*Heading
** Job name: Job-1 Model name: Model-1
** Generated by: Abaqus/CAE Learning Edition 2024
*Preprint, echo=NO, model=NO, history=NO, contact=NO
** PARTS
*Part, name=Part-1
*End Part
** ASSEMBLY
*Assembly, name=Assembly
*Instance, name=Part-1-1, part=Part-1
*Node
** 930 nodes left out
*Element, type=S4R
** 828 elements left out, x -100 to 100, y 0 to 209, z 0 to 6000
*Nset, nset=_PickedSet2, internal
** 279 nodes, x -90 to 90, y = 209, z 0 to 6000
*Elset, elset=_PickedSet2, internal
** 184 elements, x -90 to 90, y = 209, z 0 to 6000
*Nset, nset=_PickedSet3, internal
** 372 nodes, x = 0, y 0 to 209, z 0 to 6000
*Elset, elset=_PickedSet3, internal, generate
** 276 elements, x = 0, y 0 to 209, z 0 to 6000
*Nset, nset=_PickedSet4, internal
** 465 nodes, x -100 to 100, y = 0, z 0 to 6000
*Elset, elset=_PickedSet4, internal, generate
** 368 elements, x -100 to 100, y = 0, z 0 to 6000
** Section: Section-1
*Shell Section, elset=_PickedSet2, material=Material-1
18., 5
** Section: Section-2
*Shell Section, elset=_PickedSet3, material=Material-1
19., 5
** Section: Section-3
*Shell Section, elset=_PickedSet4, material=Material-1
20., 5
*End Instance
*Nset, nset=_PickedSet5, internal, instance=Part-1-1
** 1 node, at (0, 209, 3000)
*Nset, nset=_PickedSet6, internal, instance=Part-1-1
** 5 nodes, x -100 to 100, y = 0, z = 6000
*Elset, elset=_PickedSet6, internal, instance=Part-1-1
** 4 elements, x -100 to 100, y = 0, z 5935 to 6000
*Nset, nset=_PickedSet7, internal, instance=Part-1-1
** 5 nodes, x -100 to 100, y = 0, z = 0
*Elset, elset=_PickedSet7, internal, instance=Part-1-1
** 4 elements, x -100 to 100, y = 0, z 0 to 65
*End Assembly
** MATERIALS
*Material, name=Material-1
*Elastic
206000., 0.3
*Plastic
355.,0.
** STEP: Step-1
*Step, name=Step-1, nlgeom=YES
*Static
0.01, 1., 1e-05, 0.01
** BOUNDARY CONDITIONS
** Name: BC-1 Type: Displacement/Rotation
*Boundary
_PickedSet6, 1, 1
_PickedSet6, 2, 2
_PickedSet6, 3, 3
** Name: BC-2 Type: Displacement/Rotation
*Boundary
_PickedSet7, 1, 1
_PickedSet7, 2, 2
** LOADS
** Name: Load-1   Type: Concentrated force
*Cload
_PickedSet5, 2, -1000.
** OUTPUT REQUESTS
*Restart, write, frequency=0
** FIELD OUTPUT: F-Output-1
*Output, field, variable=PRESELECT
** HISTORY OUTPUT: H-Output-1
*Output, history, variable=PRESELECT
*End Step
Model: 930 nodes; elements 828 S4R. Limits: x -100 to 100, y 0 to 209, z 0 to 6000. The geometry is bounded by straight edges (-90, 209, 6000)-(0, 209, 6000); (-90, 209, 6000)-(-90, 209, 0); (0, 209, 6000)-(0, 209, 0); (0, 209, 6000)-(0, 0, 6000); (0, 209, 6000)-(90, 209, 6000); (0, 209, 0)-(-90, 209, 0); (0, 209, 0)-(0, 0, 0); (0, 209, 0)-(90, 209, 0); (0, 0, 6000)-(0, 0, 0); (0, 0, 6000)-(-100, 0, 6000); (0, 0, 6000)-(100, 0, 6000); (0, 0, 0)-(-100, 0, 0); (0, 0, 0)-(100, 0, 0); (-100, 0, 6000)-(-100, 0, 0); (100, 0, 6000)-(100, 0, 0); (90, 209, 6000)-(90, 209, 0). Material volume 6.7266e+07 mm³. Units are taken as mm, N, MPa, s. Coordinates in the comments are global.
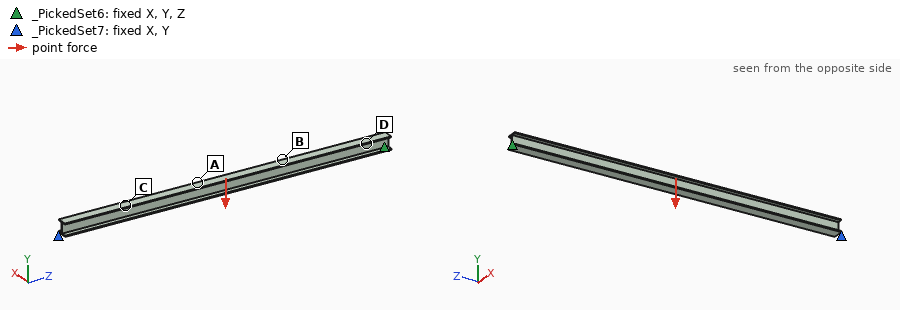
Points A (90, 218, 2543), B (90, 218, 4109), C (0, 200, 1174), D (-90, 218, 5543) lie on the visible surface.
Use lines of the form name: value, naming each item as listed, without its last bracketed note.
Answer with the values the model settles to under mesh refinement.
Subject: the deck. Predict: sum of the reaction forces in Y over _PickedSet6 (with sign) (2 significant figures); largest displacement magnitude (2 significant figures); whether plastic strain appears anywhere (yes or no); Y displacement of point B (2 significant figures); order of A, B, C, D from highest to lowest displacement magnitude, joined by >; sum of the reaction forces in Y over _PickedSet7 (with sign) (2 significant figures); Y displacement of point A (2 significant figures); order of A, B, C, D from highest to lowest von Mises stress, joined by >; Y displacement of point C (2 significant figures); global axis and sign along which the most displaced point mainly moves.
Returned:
sum of the reaction forces in Y over _PickedSet6 (with sign): 500 N
largest displacement magnitude: 0.24 mm
whether plastic strain appears anywhere: no
Y displacement of point B: -0.20 mm
order of A, B, C, D from highest to lowest displacement magnitude, joined by >: A > B > C > D
sum of the reaction forces in Y over _PickedSet7 (with sign): 500 N
Y displacement of point A: -0.23 mm
order of A, B, C, D from highest to lowest von Mises stress, joined by >: A > B > C > D
Y displacement of point C: -0.13 mm
global axis and sign along which the most displaced point mainly moves: -Y
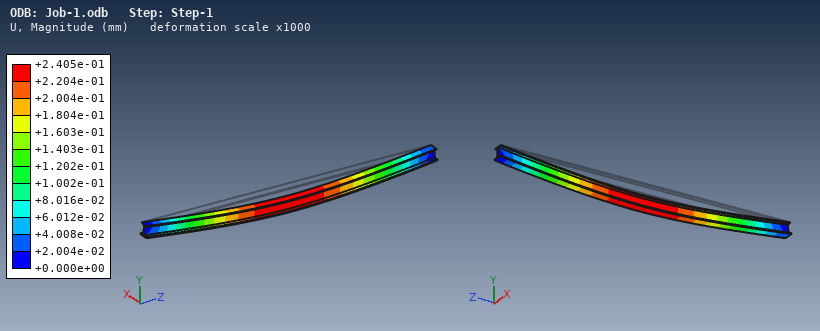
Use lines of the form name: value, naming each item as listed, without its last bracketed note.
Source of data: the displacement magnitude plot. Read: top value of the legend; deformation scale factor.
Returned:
top value of the legend: +2.405e-01 mm
deformation scale factor: 1000
